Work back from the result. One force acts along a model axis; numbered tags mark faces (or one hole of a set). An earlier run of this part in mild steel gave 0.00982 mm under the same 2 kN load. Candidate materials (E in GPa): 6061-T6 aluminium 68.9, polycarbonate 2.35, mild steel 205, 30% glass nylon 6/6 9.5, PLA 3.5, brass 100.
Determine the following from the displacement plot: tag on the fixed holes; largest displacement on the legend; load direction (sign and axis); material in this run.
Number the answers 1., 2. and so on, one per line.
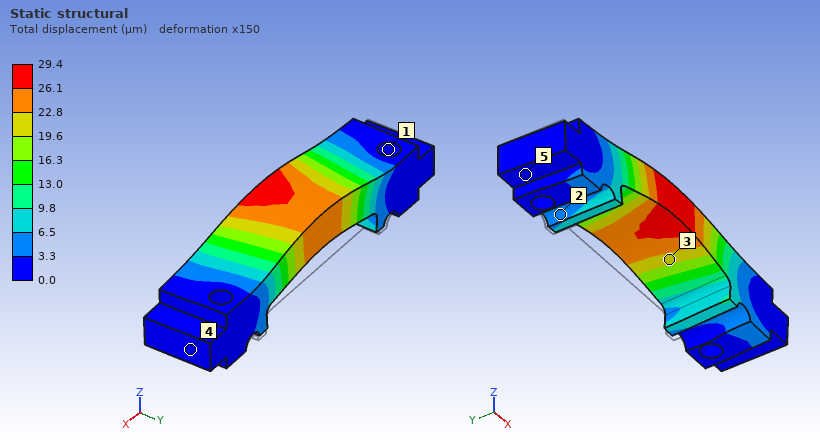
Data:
1. 1
2. 29.4 µm
3. +Z
4. 6061-T6 aluminium
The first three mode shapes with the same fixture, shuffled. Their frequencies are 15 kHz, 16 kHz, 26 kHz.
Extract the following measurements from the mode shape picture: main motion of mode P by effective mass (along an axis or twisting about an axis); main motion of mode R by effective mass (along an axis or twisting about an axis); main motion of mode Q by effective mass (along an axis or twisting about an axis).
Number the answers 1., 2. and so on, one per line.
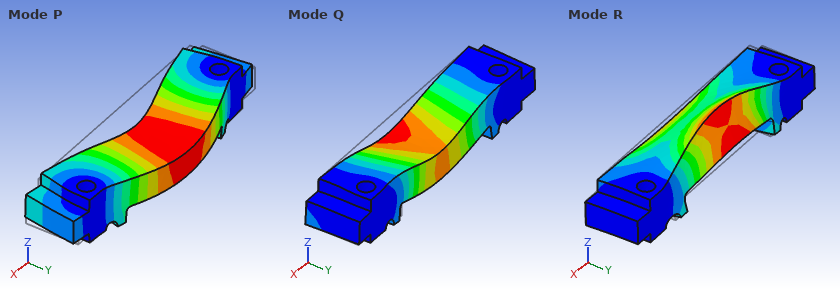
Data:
1. along Y
2. twisting about X
3. along Z
